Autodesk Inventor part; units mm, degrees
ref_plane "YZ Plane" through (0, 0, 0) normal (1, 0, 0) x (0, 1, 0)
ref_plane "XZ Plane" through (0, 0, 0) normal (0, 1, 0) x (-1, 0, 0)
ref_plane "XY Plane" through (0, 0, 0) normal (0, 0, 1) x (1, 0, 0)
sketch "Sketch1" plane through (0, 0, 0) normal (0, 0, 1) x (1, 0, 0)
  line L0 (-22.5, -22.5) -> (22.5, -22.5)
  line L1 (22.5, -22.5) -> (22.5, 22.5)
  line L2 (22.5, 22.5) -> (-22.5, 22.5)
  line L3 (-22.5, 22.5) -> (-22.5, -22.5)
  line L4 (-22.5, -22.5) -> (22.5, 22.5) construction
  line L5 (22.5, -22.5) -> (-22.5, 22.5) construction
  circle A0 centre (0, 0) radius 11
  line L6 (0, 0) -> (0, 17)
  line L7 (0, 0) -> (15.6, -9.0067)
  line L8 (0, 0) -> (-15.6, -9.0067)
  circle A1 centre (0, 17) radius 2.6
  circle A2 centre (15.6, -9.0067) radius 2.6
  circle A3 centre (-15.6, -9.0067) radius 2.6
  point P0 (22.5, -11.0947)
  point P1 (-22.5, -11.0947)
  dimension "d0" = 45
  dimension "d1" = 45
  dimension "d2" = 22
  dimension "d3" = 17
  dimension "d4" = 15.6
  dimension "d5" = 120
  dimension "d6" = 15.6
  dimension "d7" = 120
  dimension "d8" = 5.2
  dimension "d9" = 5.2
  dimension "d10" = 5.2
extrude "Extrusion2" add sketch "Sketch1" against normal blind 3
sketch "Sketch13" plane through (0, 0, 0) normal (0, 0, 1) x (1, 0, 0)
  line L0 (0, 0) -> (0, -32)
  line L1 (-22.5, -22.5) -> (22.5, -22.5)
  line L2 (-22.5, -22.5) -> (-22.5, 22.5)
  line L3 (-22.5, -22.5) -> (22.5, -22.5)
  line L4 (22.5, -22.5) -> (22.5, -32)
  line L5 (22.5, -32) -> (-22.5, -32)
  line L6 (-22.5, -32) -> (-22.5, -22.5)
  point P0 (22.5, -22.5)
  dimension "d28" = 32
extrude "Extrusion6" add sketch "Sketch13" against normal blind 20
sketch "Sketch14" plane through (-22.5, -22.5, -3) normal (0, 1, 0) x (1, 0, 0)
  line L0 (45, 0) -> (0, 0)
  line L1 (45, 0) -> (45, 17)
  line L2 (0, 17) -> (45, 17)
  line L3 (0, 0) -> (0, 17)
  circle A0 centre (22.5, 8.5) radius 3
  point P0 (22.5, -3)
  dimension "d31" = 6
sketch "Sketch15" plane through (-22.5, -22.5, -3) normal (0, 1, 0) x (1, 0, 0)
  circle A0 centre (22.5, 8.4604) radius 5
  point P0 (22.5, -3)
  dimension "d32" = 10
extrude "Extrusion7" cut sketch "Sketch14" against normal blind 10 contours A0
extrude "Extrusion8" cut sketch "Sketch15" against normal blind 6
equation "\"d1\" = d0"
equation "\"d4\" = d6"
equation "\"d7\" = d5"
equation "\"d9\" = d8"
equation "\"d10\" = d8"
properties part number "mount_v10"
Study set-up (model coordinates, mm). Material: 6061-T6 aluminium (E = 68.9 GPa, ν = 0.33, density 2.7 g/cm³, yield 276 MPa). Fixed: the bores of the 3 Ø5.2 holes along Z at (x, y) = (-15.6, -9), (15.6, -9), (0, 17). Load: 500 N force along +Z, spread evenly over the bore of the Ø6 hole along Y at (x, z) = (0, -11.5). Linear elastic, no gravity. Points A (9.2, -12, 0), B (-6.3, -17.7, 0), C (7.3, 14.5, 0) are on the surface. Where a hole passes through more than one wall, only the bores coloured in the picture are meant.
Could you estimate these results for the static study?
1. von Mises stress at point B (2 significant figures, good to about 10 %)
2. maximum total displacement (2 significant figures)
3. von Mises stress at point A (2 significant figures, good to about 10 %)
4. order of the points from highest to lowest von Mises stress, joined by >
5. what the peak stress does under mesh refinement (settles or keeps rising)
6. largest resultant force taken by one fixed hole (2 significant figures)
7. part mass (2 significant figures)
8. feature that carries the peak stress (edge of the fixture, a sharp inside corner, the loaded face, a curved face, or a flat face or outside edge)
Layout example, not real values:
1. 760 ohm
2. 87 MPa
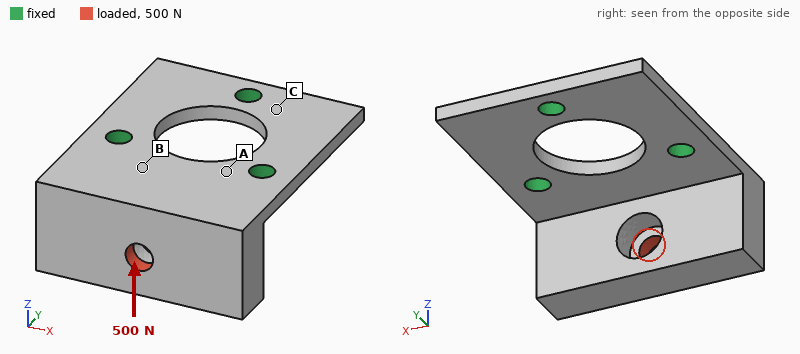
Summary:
1. 71 MPa
2. 0.36 mm
3. 110 MPa
4. A > B > C
5. keeps rising
6. 250 N
7. 34 g
8. edge of the fixture
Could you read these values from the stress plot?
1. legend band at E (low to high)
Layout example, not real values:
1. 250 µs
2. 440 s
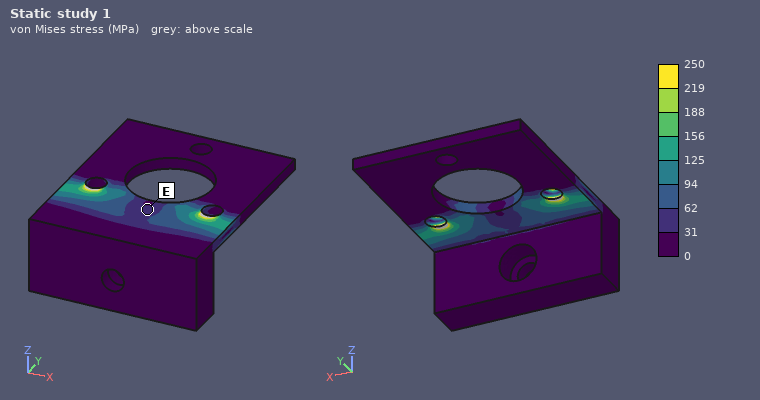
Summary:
1. 31 to 62 MPa
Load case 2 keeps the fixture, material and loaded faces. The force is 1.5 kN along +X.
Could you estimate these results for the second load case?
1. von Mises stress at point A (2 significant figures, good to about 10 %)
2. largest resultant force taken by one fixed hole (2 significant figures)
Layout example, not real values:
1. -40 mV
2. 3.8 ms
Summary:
1. 29 MPa
2. 1.2 kN
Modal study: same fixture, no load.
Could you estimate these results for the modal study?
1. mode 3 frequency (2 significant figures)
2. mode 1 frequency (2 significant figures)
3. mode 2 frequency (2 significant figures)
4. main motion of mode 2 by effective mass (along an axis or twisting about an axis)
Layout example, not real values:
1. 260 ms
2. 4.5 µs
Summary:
1. 7000 Hz
2. 1500 Hz
3. 4300 Hz
4. along X
